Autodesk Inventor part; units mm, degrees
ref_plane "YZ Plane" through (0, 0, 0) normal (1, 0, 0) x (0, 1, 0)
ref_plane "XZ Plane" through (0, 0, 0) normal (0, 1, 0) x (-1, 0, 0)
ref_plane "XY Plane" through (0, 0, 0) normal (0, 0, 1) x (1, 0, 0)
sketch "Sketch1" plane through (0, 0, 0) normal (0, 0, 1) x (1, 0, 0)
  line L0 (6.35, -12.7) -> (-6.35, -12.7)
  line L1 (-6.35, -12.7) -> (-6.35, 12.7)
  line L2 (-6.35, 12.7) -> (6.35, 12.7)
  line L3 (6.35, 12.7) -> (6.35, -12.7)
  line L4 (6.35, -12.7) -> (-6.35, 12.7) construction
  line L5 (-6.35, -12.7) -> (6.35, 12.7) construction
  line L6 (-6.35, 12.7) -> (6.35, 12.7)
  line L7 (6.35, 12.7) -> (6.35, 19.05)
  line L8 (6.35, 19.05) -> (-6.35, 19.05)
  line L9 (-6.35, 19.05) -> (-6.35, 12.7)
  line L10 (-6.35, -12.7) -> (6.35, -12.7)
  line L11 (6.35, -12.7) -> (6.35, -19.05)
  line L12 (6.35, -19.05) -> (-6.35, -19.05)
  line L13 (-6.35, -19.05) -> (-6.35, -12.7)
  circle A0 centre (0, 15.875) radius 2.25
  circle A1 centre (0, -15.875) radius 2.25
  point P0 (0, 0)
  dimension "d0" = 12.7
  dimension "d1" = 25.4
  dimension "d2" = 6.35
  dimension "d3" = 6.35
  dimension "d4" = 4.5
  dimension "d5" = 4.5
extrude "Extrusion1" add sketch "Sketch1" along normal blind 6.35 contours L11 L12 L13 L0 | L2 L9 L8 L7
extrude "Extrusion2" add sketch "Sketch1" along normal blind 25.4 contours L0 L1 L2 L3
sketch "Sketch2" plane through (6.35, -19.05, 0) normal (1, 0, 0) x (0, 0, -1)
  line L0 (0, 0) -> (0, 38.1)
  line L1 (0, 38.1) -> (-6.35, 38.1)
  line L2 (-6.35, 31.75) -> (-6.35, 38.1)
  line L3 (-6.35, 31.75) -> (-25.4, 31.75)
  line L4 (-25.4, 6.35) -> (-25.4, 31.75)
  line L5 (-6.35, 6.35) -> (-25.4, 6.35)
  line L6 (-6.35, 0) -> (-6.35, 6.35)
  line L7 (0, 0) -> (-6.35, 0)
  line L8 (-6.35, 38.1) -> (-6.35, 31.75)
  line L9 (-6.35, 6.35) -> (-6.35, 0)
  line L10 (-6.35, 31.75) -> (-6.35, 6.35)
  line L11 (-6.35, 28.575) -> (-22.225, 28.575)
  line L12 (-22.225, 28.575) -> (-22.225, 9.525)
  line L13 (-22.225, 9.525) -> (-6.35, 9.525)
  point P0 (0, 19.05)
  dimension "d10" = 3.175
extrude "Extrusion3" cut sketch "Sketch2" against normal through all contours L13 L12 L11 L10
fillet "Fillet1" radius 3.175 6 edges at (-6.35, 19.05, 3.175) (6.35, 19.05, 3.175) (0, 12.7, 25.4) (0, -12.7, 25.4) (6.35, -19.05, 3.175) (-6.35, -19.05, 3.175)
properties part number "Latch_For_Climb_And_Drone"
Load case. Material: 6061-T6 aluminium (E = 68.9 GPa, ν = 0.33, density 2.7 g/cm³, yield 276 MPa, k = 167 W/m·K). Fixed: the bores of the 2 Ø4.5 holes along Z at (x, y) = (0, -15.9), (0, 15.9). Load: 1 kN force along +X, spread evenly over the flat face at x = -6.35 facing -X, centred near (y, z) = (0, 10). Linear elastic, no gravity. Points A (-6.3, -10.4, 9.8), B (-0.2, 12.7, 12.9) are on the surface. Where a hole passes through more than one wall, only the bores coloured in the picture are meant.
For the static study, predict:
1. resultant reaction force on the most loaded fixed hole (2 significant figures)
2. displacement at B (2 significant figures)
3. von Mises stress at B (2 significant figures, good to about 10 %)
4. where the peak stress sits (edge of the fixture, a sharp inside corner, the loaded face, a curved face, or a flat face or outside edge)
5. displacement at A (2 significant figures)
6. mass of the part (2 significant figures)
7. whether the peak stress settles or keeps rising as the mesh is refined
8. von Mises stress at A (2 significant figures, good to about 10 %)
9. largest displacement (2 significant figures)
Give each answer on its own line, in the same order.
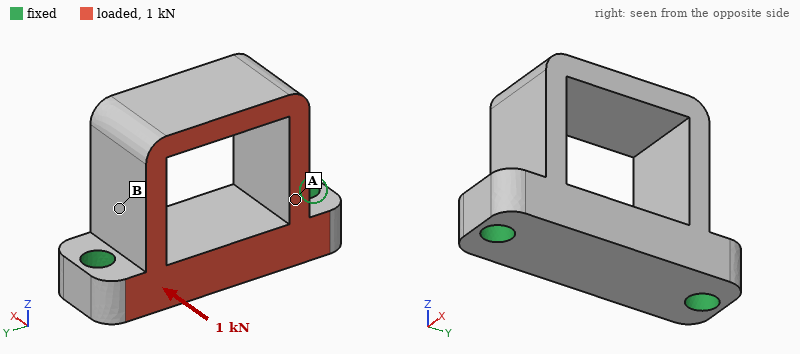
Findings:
500 N
10 µm
11 MPa
edge of the fixture
9.6 µm
14 g
keeps rising
25 MPa
30 µm
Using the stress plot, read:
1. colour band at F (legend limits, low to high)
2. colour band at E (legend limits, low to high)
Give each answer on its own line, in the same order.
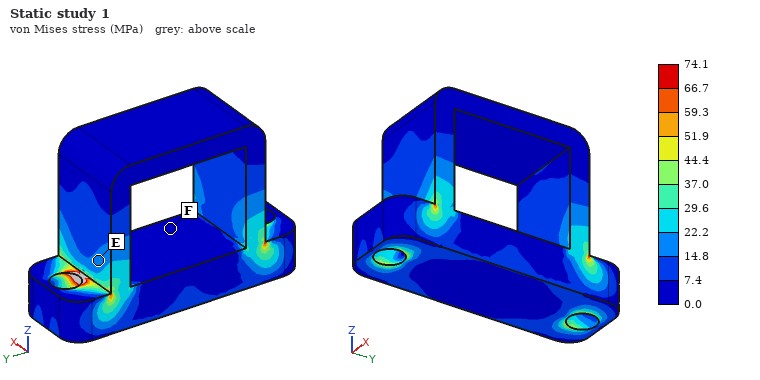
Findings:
0.0 to 7.4 MPa
14.8 to 22.2 MPa
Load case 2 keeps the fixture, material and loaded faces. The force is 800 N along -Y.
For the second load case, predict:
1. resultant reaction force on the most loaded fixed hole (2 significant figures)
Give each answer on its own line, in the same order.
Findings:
460 N
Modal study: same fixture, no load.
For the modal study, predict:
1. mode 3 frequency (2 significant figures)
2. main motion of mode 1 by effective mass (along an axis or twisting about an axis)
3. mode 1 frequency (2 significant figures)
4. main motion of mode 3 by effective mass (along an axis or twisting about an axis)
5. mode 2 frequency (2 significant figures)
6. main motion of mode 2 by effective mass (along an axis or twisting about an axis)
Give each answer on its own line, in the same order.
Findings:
14 kHz
along Y
6600 Hz
twisting about Z
9200 Hz
along X
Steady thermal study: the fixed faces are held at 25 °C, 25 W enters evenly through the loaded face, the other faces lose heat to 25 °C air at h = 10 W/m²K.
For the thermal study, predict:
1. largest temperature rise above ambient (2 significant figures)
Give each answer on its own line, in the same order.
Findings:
18 K
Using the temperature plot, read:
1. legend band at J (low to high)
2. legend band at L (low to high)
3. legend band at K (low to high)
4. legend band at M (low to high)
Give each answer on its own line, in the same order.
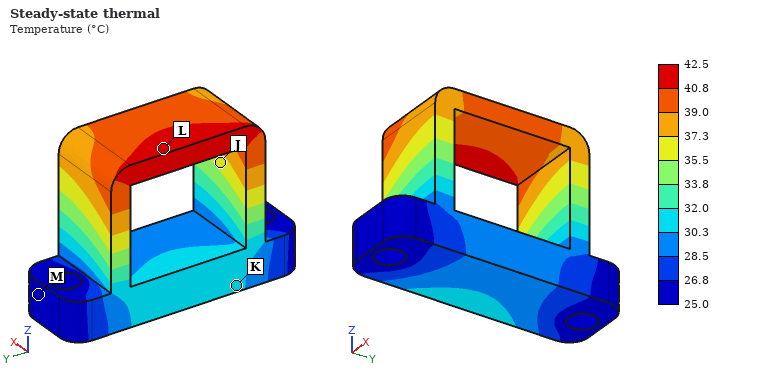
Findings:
35.5 to 37.3 °C
40.8 to 42.5 °C
30.3 to 32.0 °C
25.0 to 26.8 °C
